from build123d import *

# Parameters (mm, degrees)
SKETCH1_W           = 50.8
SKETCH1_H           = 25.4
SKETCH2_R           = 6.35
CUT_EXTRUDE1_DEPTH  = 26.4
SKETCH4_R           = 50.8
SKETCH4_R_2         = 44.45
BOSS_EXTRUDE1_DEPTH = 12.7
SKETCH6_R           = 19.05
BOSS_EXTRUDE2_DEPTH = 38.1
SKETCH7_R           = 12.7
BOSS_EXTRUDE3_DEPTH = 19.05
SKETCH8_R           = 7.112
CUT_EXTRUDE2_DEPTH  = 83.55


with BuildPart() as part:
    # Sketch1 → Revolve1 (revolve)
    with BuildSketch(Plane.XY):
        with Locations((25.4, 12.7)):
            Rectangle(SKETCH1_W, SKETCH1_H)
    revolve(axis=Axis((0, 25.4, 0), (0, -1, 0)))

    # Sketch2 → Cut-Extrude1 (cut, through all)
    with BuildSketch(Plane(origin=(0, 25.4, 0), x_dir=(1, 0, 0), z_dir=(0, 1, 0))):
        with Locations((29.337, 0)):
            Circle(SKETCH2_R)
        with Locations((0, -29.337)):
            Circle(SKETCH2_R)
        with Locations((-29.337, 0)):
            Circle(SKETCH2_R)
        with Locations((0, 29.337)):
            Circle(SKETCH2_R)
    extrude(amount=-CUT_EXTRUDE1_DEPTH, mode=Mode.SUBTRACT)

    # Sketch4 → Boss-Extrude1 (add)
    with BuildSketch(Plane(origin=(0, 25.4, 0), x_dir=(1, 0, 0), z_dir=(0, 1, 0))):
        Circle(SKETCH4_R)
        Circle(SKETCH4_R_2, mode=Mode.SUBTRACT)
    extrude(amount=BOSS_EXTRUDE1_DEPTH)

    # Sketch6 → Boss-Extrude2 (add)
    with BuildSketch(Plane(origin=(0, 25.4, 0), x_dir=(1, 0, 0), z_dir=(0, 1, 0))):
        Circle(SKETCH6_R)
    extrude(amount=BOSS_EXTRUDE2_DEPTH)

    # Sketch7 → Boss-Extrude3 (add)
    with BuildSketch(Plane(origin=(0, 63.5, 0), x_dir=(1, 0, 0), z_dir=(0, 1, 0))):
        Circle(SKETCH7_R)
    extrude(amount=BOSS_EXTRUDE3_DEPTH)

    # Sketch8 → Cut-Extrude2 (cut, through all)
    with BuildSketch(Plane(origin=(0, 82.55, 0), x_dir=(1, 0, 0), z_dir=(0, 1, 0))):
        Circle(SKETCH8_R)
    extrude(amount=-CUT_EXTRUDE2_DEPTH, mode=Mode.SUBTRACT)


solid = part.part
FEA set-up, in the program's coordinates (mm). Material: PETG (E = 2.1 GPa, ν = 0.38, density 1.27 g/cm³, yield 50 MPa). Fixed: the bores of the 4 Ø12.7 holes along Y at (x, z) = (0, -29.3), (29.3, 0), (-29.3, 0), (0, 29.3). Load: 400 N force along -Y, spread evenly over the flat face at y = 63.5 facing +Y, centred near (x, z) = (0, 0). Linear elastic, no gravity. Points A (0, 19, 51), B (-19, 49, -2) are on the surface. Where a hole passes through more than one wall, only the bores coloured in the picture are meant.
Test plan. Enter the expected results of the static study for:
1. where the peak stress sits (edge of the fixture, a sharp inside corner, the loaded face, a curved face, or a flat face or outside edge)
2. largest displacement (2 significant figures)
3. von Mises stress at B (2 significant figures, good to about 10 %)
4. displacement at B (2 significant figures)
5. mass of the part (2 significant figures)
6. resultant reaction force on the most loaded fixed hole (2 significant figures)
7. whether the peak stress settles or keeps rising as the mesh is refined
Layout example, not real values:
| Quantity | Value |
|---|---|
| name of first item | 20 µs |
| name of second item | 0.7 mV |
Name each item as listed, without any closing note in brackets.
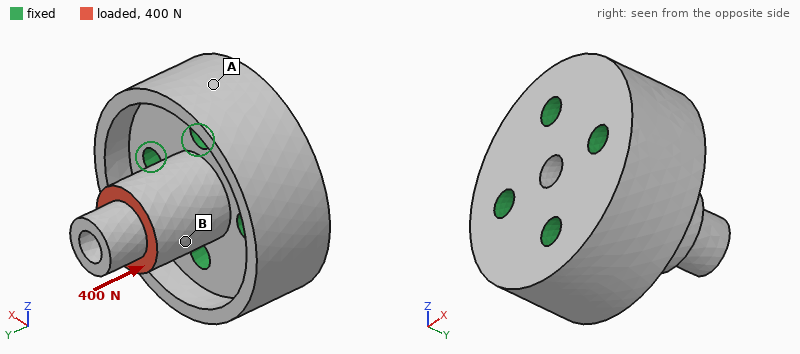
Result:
| Quantity | Value |
|---|---|
| where the peak stress sits | edge of the fixture |
| largest displacement | 11 µm |
| von Mises stress at B | 0.43 MPa |
| displacement at B | 7.3 µm |
| mass of the part | 330 g |
| resultant reaction force on the most loaded fixed hole | 110 N |
| whether the peak stress settles or keeps rising as the mesh is refined | keeps rising |
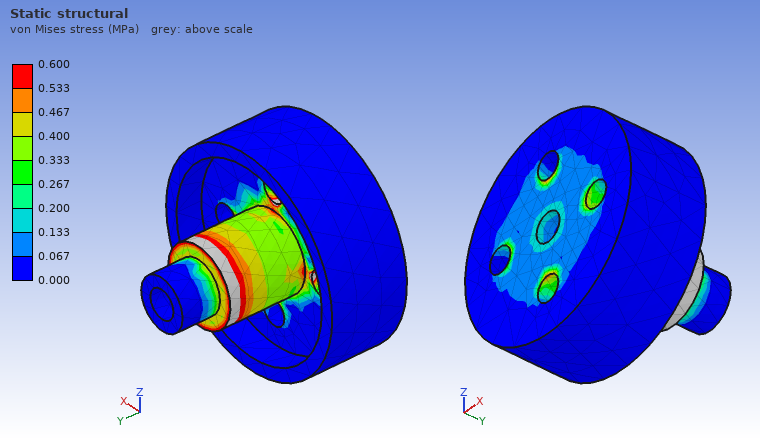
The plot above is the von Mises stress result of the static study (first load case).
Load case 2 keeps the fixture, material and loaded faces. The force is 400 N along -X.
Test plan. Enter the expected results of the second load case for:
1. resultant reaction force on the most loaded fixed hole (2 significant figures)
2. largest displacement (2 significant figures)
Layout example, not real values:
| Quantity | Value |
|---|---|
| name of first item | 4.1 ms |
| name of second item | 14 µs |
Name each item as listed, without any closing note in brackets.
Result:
| Quantity | Value |
|---|---|
| resultant reaction force on the most loaded fixed hole | 370 N |
| largest displacement | 0.12 mm |
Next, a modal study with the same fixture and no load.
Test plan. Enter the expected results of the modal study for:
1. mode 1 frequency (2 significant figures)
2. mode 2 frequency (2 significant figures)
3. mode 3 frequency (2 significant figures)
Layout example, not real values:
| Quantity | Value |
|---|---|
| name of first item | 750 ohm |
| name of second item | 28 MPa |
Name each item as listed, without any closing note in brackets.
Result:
| Quantity | Value |
|---|---|
| mode 1 frequency | 2000 Hz |
| mode 2 frequency | 2000 Hz |
| mode 3 frequency | 3900 Hz |
